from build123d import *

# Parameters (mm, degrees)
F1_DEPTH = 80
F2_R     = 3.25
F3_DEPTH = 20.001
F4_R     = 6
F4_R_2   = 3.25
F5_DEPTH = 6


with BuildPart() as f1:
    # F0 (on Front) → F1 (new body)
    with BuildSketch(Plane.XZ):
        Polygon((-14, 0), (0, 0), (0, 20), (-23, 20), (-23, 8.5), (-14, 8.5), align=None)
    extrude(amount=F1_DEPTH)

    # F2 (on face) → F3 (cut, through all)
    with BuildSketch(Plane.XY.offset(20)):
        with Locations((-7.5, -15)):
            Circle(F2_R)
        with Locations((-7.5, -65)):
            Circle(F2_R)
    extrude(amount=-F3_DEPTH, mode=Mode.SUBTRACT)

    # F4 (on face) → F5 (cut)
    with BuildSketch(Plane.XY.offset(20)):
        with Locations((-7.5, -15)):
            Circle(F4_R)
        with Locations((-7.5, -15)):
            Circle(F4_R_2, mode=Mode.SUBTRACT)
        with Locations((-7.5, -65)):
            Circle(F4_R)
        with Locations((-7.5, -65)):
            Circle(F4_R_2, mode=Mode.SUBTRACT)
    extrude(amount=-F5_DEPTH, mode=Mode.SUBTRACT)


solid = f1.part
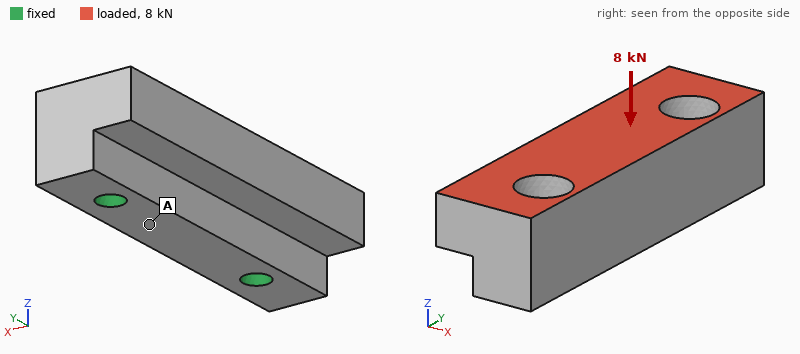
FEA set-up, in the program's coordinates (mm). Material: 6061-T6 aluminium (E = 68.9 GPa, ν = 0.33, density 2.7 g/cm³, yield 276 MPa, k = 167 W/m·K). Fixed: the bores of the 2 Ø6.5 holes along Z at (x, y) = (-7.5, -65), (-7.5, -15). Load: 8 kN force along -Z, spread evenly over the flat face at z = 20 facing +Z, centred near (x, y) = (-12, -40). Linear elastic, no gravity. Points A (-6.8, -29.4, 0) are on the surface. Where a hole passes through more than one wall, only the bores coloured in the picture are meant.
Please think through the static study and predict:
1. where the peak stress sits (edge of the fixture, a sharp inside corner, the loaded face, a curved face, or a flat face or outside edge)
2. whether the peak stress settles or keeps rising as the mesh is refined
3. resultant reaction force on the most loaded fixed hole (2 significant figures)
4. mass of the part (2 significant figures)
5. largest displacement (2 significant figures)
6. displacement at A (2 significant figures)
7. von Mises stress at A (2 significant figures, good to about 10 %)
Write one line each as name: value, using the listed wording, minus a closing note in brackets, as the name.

where the peak stress sits: edge of the fixture
whether the peak stress settles or keeps rising as the mesh is refined: keeps rising
resultant reaction force on the most loaded fixed hole: 4.1 kN
mass of the part: 77 g
largest displacement: 21 µm
displacement at A: 6.3 µm
von Mises stress at A: 9.0 MPa
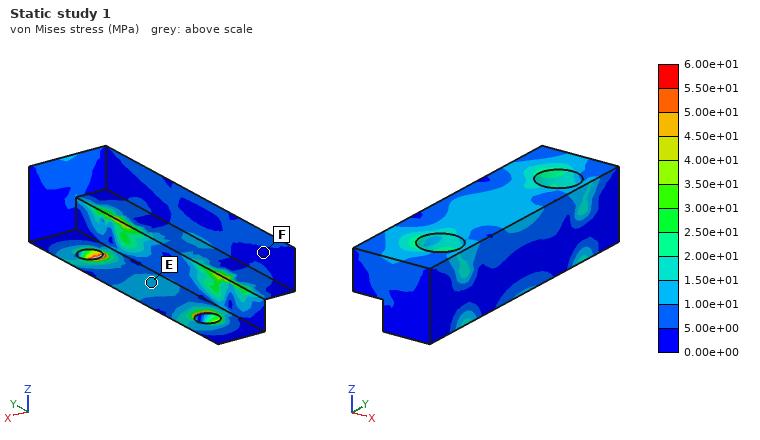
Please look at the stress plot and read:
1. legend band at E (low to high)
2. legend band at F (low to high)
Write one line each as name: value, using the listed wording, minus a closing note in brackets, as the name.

legend band at E: 1.00e+01 to 1.50e+01 MPa
legend band at F: 0.00e+00 to 5.00e+00 MPa
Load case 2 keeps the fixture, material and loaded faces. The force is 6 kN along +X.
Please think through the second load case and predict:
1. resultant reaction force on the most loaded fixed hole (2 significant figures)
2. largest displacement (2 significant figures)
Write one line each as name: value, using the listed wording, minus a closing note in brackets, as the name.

resultant reaction force on the most loaded fixed hole: 3.0 kN
largest displacement: 29 µm
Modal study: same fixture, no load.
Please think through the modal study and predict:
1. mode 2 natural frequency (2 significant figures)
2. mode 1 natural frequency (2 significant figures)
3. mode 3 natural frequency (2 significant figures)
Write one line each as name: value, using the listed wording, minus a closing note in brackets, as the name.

mode 2 natural frequency: 20 kHz
mode 1 natural frequency: 15 kHz
mode 3 natural frequency: 21 kHz
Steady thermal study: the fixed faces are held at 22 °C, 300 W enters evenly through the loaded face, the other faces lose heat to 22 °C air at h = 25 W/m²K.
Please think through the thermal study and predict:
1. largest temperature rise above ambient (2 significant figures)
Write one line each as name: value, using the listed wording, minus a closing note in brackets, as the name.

largest temperature rise above ambient: 38 K
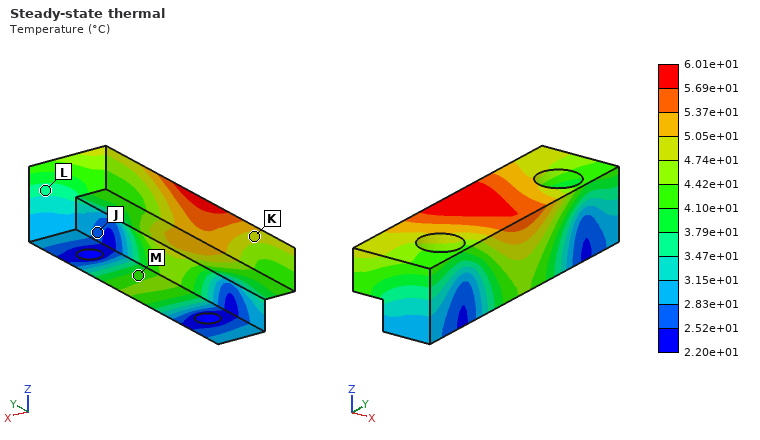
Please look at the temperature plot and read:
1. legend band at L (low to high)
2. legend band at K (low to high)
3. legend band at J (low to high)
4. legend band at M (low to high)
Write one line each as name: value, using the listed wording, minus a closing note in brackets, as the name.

legend band at L: 3.47e+01 to 3.79e+01 °C
legend band at K: 4.74e+01 to 5.05e+01 °C
legend band at J: 2.52e+01 to 2.83e+01 °C
legend band at M: 4.10e+01 to 4.42e+01 °C
